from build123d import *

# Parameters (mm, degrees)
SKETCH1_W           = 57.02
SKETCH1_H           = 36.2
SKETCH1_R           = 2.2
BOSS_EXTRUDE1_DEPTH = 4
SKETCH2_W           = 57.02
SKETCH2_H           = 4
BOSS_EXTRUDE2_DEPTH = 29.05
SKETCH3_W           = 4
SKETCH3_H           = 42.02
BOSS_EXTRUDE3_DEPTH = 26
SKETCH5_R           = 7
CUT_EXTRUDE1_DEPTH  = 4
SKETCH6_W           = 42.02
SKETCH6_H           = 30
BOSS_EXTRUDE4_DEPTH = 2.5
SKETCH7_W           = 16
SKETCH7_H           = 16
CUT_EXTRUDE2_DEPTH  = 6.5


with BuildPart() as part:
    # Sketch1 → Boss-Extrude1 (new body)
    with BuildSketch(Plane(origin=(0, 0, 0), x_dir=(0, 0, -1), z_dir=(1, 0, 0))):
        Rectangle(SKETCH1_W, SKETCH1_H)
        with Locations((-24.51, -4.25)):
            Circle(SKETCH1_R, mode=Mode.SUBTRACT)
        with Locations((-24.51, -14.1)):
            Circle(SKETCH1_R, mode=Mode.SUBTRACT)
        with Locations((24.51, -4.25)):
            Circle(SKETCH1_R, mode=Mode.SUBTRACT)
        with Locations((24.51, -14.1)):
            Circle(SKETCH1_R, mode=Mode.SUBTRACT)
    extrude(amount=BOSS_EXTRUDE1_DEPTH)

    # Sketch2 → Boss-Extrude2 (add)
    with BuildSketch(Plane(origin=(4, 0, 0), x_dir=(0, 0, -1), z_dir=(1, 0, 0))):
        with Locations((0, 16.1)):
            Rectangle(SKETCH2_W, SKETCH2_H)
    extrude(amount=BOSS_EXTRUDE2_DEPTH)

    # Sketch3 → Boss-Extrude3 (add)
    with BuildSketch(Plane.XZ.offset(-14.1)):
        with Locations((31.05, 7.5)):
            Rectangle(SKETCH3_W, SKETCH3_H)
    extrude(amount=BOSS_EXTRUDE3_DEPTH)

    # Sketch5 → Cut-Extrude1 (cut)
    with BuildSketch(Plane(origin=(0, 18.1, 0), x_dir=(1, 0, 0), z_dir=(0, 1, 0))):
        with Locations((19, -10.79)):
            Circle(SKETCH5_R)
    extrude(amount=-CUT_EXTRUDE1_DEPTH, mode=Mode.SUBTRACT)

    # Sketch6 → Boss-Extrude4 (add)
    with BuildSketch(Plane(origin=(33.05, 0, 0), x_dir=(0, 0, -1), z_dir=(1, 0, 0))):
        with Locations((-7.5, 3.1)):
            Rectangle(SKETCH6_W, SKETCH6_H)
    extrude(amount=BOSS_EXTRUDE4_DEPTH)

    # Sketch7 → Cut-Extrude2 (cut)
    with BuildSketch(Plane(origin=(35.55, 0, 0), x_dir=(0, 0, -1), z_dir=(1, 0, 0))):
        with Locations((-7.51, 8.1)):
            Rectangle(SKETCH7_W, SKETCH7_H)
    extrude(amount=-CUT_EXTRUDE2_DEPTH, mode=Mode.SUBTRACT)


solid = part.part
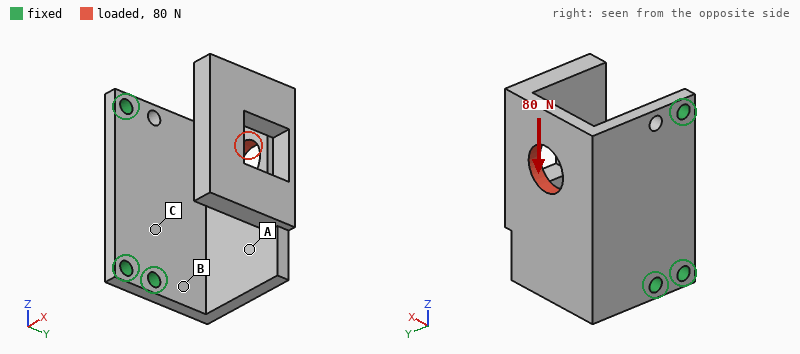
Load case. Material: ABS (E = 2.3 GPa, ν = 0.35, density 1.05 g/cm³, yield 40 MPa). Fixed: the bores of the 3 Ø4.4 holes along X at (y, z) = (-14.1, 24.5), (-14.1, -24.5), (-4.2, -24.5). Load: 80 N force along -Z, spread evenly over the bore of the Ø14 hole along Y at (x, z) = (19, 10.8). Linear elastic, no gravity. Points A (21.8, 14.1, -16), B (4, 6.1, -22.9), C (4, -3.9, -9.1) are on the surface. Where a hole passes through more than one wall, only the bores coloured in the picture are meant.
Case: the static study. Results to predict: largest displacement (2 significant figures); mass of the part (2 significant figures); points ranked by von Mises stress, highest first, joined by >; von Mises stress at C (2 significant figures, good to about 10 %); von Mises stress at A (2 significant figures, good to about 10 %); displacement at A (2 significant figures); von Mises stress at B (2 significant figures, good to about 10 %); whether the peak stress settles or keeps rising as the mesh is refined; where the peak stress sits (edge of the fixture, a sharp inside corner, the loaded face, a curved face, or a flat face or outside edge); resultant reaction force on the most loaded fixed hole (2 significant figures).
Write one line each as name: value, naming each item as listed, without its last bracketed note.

largest displacement: 0.86 mm
mass of the part: 21 g
points ranked by von Mises stress, highest first, joined by >: B > C > A
von Mises stress at C: 2.7 MPa
von Mises stress at A: 1.3 MPa
displacement at A: 0.30 mm
von Mises stress at B: 5.1 MPa
whether the peak stress settles or keeps rising as the mesh is refined: keeps rising
where the peak stress sits: edge of the fixture
resultant reaction force on the most loaded fixed hole: 58 N
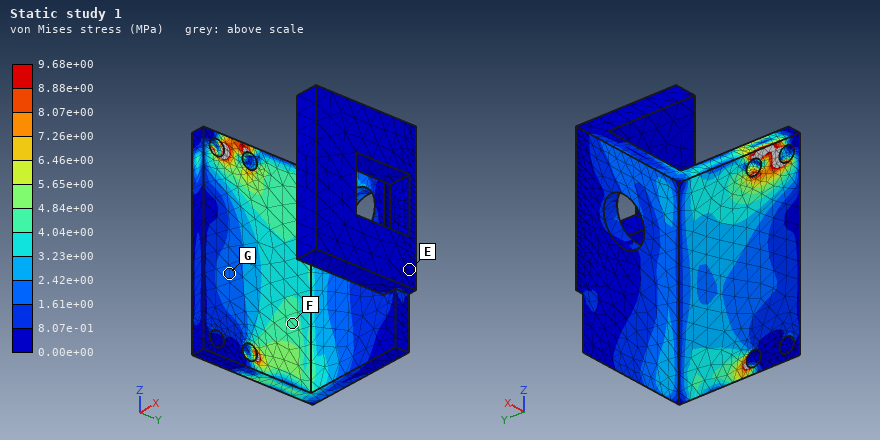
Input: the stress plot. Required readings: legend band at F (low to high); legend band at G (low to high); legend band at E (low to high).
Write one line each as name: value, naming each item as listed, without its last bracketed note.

legend band at F: 4.04e+00 to 4.84e+00 MPa
legend band at G: 1.61e+00 to 2.42e+00 MPa
legend band at E: 0.00e+00 to 8.07e-01 MPa
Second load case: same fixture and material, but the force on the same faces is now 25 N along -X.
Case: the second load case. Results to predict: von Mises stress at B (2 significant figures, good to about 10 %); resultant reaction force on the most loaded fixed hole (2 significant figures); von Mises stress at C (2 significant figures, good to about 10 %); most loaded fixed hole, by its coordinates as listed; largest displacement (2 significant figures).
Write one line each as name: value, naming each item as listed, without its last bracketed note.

von Mises stress at B: 2.9 MPa
resultant reaction force on the most loaded fixed hole: 24 N
von Mises stress at C: 2.5 MPa
most loaded fixed hole, by its coordinates as listed: (-4.2, -24.5)
largest displacement: 0.79 mm
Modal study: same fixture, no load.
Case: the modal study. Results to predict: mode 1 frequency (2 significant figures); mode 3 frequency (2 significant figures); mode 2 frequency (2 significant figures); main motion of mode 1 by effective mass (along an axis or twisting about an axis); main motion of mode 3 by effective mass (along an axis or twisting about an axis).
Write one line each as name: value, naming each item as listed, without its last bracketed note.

mode 1 frequency: 220 Hz
mode 3 frequency: 500 Hz
mode 2 frequency: 350 Hz
main motion of mode 1 by effective mass: along Y
main motion of mode 3 by effective mass: along X
